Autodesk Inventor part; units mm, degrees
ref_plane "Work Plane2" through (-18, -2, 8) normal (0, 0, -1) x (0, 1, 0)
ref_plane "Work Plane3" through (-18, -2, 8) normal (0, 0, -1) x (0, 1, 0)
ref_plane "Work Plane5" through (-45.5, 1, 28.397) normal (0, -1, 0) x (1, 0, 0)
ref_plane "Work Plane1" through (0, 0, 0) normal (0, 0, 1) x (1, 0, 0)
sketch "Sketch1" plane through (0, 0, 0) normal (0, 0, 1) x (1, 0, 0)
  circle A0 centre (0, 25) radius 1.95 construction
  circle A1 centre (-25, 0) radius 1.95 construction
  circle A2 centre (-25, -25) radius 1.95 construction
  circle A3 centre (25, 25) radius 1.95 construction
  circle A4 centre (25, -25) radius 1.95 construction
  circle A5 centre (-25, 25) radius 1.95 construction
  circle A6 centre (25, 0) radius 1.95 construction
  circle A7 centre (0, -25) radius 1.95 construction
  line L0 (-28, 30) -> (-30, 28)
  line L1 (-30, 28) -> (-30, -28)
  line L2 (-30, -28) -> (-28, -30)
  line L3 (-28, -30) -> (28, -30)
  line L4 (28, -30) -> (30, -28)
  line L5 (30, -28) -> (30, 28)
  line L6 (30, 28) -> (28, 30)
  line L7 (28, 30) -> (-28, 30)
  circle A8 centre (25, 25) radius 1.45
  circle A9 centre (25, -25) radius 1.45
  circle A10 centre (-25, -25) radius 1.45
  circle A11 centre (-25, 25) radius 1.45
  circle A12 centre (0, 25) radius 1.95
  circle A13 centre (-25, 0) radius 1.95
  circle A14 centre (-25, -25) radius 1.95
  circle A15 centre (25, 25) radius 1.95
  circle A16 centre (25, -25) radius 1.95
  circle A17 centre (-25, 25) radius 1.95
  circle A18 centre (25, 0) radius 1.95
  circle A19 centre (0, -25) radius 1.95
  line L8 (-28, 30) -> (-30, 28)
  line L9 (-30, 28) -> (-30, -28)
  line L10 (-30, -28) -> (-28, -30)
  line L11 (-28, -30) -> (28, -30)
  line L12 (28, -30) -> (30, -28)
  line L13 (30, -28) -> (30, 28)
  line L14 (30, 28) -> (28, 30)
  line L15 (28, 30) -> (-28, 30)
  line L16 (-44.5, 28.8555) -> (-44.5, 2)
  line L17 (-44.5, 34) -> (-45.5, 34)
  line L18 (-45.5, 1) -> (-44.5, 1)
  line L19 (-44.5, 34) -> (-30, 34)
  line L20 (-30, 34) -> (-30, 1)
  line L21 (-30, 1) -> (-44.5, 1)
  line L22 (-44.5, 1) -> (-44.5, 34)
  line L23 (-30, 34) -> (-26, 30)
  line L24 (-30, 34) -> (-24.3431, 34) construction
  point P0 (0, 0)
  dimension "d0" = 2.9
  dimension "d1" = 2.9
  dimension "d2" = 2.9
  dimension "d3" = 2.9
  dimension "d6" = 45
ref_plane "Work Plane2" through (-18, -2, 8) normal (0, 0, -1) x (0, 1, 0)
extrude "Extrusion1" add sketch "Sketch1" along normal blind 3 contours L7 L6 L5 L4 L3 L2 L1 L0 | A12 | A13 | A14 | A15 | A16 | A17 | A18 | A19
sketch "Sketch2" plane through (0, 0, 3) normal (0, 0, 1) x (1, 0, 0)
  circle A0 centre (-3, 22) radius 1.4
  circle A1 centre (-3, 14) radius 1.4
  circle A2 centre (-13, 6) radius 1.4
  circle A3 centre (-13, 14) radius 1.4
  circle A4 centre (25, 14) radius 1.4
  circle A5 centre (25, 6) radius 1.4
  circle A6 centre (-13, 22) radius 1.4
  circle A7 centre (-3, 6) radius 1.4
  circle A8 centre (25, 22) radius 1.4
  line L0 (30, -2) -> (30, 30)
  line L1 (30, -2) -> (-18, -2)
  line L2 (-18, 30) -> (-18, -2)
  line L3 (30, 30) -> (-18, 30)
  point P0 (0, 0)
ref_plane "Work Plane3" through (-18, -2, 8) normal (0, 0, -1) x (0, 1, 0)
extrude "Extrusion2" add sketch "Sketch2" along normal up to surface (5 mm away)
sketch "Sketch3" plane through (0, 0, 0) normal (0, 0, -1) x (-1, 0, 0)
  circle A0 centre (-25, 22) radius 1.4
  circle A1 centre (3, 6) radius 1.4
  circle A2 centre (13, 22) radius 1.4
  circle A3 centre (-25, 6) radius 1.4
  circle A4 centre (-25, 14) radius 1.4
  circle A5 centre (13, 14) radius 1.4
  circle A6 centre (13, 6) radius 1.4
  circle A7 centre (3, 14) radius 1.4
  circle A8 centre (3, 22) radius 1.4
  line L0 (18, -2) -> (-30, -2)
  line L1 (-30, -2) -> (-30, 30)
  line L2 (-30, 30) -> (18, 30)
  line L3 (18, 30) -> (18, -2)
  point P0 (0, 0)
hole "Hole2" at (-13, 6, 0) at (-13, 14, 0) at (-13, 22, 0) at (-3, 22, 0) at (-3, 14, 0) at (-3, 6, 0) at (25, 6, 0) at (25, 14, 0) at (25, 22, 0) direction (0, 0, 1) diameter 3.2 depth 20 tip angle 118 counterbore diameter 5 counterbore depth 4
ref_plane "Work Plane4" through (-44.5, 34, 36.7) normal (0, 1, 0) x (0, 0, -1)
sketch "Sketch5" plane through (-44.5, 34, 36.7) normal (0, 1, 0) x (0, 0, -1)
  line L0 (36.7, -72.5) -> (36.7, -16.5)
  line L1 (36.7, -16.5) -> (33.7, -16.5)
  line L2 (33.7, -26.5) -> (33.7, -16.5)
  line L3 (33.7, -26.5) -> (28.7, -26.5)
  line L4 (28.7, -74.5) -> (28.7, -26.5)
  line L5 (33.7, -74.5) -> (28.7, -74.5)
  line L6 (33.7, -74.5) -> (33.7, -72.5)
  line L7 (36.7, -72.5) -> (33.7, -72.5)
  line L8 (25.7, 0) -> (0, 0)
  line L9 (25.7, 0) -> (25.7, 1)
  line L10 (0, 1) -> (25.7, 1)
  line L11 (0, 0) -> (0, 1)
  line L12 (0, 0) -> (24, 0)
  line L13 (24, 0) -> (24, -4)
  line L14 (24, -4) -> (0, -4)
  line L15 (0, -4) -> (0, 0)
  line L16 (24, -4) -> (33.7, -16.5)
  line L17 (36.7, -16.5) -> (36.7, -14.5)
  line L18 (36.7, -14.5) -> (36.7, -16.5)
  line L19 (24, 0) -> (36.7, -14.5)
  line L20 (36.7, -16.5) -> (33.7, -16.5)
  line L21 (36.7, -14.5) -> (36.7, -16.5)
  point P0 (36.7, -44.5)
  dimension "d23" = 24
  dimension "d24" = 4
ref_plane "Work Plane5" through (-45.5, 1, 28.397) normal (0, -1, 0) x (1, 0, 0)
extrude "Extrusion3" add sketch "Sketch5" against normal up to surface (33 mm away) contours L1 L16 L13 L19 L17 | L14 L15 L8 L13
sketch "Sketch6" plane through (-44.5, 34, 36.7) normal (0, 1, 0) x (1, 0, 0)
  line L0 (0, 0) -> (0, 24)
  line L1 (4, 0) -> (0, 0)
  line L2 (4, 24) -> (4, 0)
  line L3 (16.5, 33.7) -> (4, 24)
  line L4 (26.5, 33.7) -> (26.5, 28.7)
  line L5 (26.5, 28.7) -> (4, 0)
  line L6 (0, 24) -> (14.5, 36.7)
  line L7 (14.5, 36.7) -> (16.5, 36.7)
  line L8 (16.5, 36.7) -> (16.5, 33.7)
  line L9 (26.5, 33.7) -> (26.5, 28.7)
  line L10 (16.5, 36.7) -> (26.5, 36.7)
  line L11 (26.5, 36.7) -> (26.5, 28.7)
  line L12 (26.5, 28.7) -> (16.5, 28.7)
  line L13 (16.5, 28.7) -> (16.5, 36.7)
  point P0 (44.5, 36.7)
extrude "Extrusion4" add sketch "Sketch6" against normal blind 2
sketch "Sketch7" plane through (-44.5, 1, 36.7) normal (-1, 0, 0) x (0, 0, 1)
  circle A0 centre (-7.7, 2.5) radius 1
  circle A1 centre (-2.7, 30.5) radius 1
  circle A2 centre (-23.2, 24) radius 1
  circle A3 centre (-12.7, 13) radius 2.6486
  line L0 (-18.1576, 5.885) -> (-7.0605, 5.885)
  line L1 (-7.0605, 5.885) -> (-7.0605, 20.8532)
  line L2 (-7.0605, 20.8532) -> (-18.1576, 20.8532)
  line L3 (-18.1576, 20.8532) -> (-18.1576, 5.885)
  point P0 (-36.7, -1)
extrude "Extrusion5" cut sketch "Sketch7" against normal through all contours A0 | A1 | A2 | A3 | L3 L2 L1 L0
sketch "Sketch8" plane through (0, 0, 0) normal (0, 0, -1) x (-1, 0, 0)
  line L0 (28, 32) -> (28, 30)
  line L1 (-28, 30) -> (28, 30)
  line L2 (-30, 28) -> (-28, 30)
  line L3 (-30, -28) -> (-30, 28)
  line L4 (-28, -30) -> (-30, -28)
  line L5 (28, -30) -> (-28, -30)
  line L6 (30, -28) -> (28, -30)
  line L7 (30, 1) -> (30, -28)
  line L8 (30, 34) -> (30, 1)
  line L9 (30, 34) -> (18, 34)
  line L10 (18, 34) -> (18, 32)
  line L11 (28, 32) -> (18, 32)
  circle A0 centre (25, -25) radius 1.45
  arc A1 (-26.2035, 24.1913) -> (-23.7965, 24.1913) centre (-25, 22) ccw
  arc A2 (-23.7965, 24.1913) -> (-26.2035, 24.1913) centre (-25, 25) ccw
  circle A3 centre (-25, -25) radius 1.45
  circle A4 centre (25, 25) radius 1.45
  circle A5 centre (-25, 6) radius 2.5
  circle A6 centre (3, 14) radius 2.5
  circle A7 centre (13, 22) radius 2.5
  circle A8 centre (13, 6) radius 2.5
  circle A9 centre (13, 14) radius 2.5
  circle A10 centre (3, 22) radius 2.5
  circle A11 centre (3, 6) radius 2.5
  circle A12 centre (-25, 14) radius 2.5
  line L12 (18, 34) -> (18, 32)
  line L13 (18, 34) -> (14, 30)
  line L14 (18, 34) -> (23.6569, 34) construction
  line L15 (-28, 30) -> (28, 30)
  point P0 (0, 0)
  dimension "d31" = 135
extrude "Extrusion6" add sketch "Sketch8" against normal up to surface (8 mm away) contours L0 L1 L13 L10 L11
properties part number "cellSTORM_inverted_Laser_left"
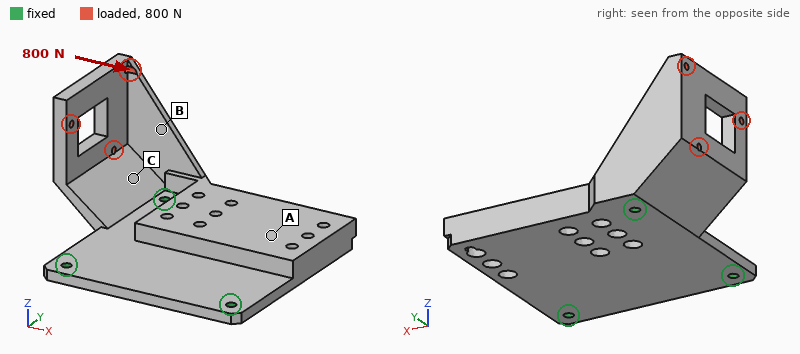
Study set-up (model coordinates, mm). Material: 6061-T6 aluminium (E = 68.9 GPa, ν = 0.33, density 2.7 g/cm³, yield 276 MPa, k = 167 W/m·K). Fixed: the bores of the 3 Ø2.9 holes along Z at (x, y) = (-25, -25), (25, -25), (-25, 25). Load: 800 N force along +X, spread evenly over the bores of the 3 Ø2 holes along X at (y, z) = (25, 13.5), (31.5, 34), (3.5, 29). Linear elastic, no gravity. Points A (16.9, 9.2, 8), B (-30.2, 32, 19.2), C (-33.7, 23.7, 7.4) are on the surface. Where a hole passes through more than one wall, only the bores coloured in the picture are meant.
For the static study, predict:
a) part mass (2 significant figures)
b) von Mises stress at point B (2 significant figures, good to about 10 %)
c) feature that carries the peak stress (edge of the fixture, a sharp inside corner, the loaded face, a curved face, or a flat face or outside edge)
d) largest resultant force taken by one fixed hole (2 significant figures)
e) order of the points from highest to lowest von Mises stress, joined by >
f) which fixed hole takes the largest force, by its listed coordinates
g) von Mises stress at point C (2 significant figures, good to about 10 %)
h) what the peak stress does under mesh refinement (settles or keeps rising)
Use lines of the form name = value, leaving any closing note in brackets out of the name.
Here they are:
part mass = 61 g
von Mises stress at point B = 80 MPa
feature that carries the peak stress = edge of the fixture
largest resultant force taken by one fixed hole = 760 N
order of the points from highest to lowest von Mises stress, joined by > = B > C > A
which fixed hole takes the largest force, by its listed coordinates = (25, -25)
von Mises stress at point C = 42 MPa
what the peak stress does under mesh refinement = keeps rising
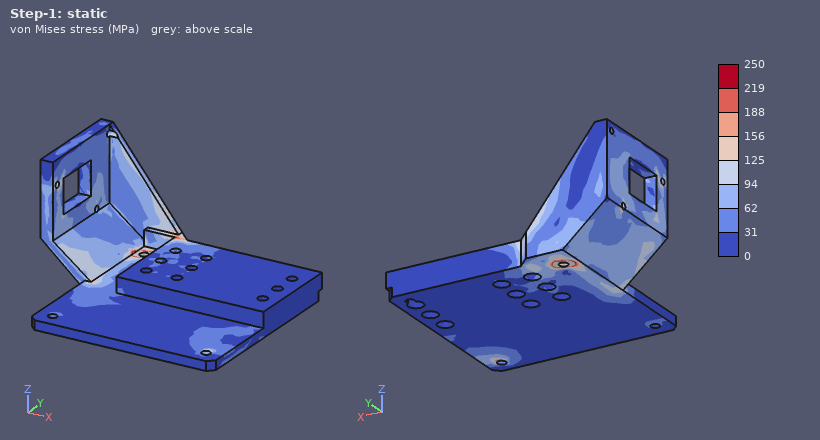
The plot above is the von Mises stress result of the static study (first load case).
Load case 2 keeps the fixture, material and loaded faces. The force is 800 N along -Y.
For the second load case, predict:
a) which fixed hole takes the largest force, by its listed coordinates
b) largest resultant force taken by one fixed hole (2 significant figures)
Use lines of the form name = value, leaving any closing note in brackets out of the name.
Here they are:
which fixed hole takes the largest force, by its listed coordinates = (-25, 25)
largest resultant force taken by one fixed hole = 730 N
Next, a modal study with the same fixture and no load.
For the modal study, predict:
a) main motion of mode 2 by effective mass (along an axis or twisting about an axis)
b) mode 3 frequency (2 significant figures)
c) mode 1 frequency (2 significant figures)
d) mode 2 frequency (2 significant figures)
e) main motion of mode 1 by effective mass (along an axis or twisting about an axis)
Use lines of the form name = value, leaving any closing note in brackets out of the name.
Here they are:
main motion of mode 2 by effective mass = along Z
mode 3 frequency = 2700 Hz
mode 1 frequency = 1500 Hz
mode 2 frequency = 2200 Hz
main motion of mode 1 by effective mass = along Z
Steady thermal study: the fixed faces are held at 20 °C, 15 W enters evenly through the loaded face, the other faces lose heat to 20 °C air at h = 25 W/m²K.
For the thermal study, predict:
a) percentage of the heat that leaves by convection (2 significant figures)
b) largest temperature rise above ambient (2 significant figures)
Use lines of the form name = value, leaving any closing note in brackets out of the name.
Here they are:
percentage of the heat that leaves by convection = 15 %
largest temperature rise above ambient = 31 K
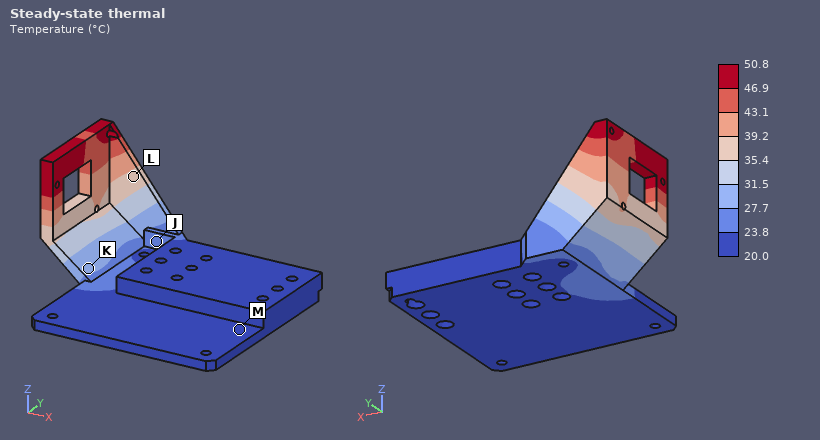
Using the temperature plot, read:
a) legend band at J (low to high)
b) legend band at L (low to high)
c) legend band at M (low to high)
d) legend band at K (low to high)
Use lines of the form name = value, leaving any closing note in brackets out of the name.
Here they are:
legend band at J = 23.8 to 27.7 °C
legend band at L = 35.4 to 39.2 °C
legend band at M = 20.0 to 23.8 °C
legend band at K = 27.7 to 31.5 °C
